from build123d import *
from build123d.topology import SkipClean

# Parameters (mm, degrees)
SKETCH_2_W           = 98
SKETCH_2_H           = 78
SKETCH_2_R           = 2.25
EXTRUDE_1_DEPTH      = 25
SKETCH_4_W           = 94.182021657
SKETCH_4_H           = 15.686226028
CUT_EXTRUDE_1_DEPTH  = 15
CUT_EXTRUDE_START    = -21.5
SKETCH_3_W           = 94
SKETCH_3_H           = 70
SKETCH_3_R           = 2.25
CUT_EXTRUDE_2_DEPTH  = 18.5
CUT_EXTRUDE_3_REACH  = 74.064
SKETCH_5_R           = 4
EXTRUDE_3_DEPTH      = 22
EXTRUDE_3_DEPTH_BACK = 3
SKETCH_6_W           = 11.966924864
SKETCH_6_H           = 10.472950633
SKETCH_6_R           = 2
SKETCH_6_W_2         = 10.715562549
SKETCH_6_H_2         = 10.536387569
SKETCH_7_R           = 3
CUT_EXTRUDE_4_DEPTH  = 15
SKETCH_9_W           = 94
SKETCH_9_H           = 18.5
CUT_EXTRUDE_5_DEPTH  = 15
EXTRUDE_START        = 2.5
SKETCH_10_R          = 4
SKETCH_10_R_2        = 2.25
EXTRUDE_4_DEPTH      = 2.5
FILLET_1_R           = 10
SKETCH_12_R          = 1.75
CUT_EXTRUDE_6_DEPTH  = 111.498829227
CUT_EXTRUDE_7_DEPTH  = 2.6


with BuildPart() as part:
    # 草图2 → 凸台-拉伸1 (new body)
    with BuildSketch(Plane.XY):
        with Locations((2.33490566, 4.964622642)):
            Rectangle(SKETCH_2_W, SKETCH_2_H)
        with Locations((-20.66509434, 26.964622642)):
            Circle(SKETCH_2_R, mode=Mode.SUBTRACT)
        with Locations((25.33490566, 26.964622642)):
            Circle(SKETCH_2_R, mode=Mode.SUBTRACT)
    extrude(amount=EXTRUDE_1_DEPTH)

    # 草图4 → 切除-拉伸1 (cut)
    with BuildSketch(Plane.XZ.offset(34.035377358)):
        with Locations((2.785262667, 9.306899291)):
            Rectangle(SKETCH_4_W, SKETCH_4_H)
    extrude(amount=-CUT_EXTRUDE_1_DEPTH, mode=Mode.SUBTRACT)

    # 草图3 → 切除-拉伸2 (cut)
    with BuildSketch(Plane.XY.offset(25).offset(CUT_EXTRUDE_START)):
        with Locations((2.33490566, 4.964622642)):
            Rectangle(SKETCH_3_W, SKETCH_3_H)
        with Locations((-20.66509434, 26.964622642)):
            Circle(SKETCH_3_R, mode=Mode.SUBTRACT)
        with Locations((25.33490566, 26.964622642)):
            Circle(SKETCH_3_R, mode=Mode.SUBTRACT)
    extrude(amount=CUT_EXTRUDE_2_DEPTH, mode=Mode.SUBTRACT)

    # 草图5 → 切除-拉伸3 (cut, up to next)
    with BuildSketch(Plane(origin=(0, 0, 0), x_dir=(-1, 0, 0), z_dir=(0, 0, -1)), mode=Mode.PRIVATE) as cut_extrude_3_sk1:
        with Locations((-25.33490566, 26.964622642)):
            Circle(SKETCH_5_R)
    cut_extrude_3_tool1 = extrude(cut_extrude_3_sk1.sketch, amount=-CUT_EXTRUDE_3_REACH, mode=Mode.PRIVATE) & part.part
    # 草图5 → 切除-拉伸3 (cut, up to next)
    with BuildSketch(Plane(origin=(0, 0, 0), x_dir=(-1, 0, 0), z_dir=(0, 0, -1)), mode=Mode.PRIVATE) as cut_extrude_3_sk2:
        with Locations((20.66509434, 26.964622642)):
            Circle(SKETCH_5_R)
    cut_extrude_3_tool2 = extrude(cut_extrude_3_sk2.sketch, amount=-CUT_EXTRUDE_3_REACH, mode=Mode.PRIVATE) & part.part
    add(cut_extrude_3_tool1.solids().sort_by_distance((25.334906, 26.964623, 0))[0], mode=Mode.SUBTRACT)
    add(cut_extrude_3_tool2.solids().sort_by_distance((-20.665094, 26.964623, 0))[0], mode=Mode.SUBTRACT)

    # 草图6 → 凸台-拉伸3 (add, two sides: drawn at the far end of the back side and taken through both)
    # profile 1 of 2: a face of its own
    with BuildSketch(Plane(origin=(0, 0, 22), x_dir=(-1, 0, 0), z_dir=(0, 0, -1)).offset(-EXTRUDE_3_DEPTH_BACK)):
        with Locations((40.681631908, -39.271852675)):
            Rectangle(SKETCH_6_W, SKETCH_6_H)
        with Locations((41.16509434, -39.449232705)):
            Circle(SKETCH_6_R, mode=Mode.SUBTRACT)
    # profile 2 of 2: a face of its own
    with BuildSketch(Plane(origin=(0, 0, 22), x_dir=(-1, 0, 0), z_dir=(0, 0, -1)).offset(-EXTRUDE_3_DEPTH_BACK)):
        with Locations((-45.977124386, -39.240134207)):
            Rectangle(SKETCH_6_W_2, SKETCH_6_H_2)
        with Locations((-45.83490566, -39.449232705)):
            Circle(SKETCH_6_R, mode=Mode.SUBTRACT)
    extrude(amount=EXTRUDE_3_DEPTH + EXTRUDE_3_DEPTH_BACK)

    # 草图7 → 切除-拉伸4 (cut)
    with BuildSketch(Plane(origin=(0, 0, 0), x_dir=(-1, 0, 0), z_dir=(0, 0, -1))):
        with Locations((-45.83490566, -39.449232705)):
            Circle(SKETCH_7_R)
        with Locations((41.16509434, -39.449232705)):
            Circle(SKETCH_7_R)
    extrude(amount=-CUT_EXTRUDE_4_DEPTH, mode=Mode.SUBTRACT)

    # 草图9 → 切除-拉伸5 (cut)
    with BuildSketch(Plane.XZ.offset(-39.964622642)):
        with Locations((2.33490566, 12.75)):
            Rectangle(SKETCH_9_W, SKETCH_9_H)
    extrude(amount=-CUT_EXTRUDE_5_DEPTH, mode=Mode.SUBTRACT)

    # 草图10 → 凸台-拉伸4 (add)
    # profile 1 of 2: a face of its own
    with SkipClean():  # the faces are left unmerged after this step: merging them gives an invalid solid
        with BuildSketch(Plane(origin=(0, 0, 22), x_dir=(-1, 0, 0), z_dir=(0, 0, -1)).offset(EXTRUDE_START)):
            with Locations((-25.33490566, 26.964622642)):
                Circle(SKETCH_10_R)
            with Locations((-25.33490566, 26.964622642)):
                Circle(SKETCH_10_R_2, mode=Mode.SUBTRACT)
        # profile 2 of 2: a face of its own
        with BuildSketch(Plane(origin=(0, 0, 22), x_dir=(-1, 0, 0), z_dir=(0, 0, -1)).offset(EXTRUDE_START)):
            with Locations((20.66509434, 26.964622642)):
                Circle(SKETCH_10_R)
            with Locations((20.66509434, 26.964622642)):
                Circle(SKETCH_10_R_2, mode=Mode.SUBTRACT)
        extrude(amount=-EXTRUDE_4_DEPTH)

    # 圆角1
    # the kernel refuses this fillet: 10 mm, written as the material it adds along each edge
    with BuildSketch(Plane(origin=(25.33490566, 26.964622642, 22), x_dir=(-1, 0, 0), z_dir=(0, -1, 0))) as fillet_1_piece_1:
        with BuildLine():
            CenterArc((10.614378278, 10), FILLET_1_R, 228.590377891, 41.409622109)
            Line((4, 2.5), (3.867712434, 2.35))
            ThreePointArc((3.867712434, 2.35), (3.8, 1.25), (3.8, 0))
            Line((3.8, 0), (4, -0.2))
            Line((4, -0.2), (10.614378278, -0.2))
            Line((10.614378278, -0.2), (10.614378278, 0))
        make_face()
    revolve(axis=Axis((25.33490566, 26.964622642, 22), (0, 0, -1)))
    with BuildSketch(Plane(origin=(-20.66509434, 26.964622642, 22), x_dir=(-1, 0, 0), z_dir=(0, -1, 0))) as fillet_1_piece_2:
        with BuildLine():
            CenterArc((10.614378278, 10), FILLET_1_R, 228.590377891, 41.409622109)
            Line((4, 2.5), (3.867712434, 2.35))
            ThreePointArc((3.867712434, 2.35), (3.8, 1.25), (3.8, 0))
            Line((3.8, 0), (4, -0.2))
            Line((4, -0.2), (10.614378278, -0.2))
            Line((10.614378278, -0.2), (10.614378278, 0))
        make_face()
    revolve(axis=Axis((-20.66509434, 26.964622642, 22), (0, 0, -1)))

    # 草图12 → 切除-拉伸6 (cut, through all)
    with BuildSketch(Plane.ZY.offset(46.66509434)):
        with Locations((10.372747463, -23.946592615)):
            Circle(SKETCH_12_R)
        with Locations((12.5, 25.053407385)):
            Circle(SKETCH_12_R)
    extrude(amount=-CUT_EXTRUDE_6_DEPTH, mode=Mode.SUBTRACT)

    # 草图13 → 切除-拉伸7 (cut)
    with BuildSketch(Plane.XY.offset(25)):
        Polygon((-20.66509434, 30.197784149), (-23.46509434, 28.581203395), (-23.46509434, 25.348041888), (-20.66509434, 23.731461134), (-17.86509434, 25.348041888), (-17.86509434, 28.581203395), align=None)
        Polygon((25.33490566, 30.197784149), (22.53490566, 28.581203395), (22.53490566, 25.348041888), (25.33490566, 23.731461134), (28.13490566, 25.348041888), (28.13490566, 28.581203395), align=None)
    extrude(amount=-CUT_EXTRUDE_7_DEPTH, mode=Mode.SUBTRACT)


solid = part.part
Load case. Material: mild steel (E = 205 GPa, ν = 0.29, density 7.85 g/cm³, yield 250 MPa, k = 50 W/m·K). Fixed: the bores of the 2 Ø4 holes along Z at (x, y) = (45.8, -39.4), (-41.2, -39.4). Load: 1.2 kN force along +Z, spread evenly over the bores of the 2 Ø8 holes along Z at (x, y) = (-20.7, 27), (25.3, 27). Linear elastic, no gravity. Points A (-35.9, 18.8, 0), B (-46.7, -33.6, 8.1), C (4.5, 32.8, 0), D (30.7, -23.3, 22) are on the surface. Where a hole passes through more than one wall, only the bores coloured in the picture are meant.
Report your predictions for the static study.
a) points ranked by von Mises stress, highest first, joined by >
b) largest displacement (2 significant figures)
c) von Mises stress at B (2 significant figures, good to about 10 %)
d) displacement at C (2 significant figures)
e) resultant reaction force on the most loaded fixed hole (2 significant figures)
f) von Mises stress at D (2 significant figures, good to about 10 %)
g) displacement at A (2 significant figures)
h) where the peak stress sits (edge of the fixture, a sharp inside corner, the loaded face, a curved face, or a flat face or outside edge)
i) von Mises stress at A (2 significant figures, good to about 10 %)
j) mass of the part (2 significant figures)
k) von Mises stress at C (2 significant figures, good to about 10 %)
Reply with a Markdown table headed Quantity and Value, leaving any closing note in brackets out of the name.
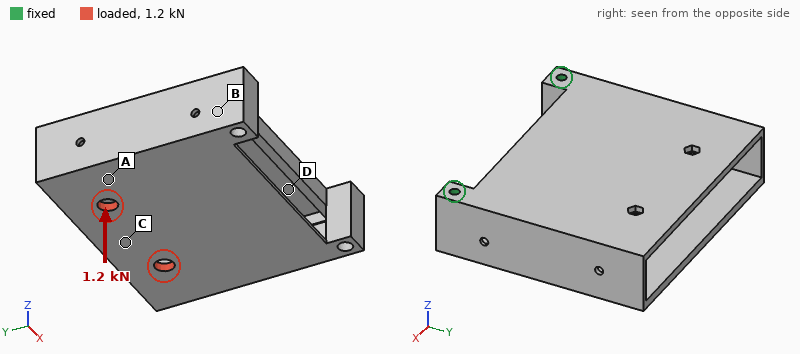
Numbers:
| Quantity | Value |
|---|---|
| points ranked by von Mises stress, highest first, joined by > | C > A > B > D |
| largest displacement | 0.36 mm |
| von Mises stress at B | 25 MPa |
| displacement at C | 0.31 mm |
| resultant reaction force on the most loaded fixed hole | 630 N |
| von Mises stress at D | 14 MPa |
| displacement at A | 0.13 mm |
| where the peak stress sits | edge of the fixture |
| von Mises stress at A | 48 MPa |
| mass of the part | 460 g |
| von Mises stress at C | 67 MPa |
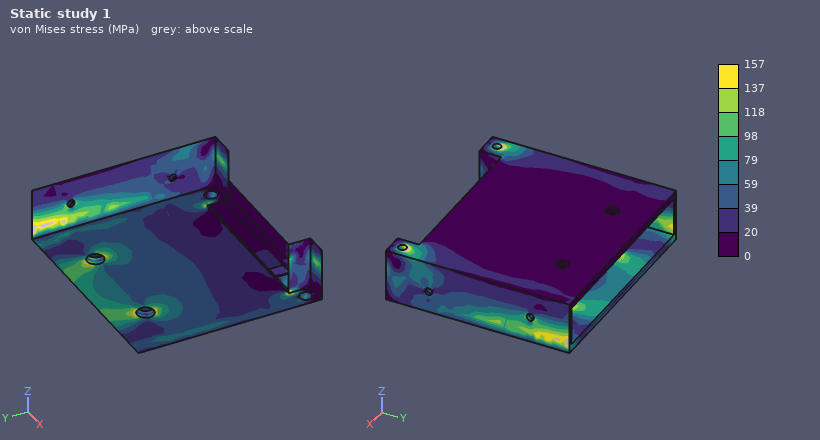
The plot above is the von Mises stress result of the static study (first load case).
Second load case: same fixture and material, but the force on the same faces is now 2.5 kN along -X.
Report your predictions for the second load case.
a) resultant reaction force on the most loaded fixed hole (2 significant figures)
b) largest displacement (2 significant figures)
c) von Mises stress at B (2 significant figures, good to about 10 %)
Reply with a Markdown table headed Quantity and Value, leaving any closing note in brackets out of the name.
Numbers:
| Quantity | Value |
|---|---|
| resultant reaction force on the most loaded fixed hole | 2.2 kN |
| largest displacement | 69 µm |
| von Mises stress at B | 42 MPa |
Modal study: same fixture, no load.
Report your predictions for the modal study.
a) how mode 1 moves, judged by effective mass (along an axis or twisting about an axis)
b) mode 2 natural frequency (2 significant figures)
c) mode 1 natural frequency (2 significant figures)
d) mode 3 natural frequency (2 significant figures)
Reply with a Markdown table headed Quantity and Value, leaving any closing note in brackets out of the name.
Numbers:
| Quantity | Value |
|---|---|
| how mode 1 moves, judged by effective mass | along Z |
| mode 2 natural frequency | 1300 Hz |
| mode 1 natural frequency | 960 Hz |
| mode 3 natural frequency | 1700 Hz |
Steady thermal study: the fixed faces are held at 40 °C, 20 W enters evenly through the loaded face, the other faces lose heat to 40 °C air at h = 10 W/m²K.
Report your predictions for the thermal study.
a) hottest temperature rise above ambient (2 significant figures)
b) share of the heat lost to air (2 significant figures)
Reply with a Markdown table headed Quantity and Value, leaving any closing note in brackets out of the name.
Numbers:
| Quantity | Value |
|---|---|
| hottest temperature rise above ambient | 67 K |
| share of the heat lost to air | 54 % |
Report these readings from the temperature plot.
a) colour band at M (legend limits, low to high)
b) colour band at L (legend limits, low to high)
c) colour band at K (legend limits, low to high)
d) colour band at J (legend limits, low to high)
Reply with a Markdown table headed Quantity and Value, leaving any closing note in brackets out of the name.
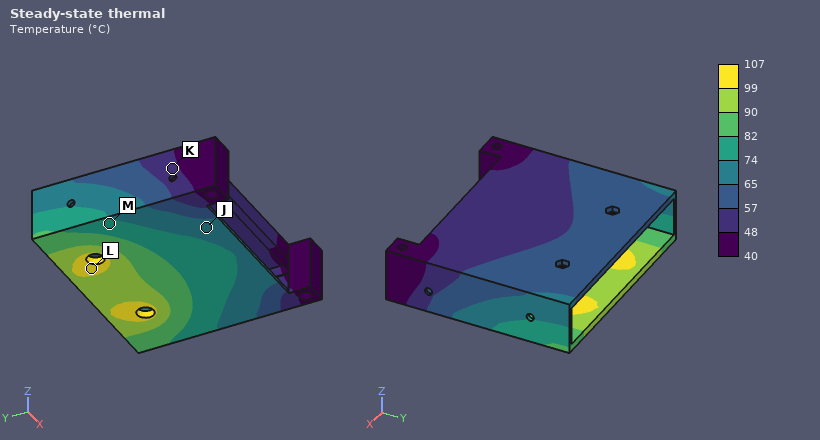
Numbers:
| Quantity | Value |
|---|---|
| colour band at M | 74 to 82 °C |
| colour band at L | 99 to 107 °C |
| colour band at K | 48 to 57 °C |
| colour band at J | 65 to 74 °C |
